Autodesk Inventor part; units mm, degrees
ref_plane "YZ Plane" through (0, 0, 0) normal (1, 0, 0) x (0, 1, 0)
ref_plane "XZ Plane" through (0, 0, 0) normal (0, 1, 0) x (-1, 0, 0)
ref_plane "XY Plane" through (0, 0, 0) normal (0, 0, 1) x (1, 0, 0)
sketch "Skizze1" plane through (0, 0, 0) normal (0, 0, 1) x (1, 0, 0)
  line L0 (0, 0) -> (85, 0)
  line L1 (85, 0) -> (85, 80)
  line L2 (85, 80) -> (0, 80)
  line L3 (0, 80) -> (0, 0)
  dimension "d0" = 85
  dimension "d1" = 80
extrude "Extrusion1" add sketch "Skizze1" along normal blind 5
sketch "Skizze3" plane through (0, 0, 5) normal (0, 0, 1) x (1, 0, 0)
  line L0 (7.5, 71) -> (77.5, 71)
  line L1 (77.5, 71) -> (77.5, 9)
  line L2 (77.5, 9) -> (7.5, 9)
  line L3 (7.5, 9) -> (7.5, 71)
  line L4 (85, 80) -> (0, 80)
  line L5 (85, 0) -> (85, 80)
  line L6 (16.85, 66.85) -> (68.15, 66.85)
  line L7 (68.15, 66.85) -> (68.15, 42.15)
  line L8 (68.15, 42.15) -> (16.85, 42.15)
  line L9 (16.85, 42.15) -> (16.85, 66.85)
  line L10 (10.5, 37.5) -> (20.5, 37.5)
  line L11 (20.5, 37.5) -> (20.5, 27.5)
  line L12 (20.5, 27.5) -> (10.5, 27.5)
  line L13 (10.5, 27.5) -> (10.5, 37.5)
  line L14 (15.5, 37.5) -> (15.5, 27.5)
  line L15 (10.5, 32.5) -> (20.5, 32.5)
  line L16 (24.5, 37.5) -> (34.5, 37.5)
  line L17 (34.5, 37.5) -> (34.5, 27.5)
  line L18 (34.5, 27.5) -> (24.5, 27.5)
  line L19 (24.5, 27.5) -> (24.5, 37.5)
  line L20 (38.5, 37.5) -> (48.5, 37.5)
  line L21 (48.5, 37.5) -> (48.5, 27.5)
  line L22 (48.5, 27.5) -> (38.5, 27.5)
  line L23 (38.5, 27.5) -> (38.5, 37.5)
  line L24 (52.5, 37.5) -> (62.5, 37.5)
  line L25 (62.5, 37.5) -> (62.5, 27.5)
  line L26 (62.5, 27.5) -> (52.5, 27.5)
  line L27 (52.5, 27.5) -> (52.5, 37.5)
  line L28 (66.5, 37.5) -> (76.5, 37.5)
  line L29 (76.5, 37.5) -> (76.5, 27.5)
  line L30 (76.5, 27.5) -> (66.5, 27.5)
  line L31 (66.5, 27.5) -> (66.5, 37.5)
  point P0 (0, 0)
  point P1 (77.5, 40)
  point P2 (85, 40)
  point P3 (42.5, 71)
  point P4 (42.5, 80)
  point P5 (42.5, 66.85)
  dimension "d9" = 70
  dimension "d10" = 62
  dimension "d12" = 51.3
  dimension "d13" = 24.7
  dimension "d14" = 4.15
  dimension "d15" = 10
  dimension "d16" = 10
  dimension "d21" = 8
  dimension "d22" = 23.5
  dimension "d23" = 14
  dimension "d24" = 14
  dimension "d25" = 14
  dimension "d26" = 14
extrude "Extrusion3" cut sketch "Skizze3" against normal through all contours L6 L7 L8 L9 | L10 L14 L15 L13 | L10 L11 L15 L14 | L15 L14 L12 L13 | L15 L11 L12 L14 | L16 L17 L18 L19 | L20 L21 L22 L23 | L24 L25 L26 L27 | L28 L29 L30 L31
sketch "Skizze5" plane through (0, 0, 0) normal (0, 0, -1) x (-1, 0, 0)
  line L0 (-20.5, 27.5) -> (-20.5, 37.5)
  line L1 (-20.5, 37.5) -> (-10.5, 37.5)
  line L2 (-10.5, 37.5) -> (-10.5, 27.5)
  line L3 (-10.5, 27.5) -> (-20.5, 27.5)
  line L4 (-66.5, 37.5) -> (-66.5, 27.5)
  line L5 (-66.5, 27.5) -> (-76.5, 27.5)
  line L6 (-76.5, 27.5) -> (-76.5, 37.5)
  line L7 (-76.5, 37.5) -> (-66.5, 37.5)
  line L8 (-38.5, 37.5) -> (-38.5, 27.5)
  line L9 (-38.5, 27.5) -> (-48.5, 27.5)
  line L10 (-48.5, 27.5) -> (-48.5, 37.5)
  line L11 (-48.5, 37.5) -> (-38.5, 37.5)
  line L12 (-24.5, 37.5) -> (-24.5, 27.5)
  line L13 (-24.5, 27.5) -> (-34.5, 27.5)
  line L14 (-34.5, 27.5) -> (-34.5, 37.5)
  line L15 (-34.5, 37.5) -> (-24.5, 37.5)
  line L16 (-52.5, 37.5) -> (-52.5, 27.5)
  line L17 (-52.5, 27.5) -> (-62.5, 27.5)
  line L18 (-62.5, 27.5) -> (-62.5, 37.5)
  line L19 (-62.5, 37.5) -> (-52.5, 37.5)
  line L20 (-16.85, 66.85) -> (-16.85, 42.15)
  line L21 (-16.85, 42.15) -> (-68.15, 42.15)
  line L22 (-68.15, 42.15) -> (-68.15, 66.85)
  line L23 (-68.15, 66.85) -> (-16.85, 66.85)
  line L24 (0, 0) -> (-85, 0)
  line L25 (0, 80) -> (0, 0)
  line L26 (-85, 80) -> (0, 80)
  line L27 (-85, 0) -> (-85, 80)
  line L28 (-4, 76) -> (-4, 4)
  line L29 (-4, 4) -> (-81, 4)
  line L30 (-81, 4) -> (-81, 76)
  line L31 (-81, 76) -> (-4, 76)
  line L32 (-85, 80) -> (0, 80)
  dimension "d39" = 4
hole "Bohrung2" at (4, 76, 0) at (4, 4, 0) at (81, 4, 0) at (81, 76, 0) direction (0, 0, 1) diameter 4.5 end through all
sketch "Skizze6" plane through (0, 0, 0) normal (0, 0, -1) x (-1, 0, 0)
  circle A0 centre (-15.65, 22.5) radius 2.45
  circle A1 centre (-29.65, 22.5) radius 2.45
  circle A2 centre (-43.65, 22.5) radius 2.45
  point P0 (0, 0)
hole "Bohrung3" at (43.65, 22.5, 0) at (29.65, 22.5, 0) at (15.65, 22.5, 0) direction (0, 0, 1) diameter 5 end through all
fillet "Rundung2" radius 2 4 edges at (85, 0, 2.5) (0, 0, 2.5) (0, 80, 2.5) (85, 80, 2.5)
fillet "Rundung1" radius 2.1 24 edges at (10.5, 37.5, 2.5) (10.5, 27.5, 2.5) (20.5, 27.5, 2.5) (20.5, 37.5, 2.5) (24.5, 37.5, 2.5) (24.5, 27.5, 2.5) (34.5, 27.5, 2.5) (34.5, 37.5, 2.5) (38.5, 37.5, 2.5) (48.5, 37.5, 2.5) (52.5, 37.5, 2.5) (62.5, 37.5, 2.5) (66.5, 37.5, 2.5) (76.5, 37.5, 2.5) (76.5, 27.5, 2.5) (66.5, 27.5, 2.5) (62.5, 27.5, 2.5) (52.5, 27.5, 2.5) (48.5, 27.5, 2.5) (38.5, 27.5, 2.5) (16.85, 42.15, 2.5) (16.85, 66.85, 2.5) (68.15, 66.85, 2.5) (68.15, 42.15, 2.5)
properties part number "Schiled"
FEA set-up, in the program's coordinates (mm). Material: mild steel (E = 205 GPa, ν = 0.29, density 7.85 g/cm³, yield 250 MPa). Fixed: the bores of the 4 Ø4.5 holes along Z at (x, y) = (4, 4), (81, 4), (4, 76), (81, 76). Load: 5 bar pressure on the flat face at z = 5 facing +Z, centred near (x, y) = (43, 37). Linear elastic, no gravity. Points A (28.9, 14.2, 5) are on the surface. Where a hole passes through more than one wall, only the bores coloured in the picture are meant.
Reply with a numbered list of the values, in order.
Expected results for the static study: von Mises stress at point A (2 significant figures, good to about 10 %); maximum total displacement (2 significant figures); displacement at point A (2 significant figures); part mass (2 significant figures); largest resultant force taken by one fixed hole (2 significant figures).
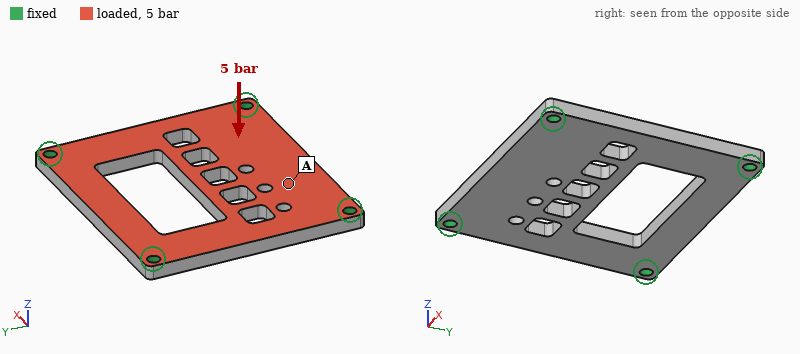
1. 27 MPa
2. 70 µm
3. 34 µm
4. 190 g
5. 680 N
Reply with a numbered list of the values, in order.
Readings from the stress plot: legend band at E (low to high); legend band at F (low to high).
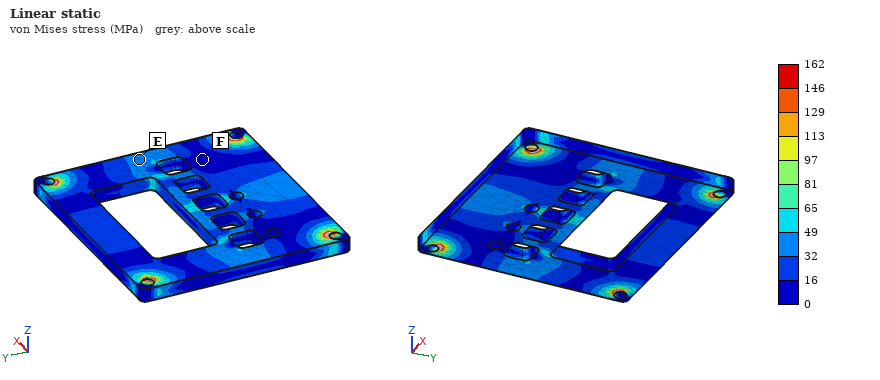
1. 32 to 49 MPa
2. 0 to 16 MPa
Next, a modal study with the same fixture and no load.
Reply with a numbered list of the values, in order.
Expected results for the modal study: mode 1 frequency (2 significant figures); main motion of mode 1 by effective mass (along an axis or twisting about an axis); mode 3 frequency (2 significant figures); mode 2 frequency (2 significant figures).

1. 3000 Hz
2. along Z
3. 5100 Hz
4. 4700 Hz
